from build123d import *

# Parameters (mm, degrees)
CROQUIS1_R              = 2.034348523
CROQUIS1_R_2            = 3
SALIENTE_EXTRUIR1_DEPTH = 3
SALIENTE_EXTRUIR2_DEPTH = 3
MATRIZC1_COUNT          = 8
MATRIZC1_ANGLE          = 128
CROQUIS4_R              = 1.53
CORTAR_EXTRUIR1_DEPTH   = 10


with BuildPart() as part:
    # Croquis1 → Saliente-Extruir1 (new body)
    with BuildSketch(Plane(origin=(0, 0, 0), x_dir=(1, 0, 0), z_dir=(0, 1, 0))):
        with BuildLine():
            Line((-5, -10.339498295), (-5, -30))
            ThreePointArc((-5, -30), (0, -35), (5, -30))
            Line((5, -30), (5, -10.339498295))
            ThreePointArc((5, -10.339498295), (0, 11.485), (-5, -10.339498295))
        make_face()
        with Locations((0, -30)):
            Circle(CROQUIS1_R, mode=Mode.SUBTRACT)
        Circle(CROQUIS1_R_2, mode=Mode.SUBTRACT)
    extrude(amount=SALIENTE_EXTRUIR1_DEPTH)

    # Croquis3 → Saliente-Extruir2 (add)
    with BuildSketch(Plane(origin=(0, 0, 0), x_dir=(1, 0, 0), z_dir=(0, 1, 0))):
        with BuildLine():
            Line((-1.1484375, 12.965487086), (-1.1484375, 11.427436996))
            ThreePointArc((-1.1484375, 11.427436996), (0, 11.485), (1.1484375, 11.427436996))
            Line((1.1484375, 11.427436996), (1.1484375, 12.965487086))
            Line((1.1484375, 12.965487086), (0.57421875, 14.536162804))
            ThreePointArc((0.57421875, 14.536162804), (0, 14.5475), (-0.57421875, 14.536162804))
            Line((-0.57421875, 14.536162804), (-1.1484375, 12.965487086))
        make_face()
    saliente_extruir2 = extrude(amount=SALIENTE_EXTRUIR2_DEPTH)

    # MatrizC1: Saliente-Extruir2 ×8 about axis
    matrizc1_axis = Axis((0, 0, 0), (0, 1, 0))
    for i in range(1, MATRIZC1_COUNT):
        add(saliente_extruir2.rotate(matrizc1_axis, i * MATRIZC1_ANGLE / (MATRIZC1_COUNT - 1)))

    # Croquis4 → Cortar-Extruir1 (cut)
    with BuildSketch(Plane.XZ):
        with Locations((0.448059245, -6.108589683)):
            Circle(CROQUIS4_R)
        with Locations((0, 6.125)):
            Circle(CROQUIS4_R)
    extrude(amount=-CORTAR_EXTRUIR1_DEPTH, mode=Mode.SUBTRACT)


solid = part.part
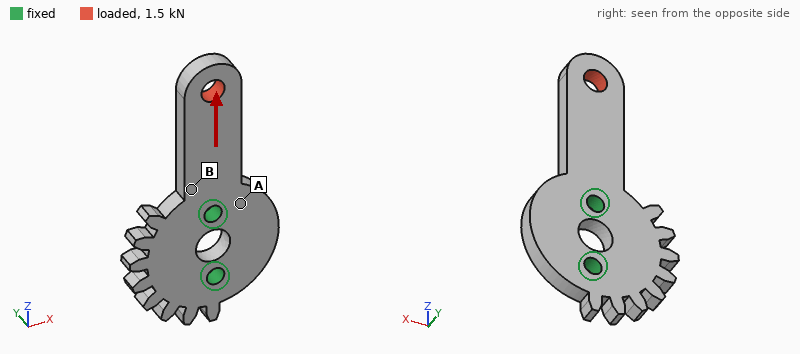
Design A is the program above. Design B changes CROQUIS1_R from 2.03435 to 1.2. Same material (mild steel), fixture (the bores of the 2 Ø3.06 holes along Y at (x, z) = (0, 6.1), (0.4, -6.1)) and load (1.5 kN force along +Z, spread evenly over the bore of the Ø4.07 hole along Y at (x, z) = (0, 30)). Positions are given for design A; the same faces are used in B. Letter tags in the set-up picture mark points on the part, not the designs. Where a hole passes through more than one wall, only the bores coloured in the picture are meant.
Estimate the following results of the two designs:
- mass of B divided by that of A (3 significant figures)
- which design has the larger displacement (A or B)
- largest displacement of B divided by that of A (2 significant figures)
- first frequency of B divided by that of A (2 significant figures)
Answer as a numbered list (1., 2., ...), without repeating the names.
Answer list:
1. 1.01
2. A
3. 0.91
4. 0.96
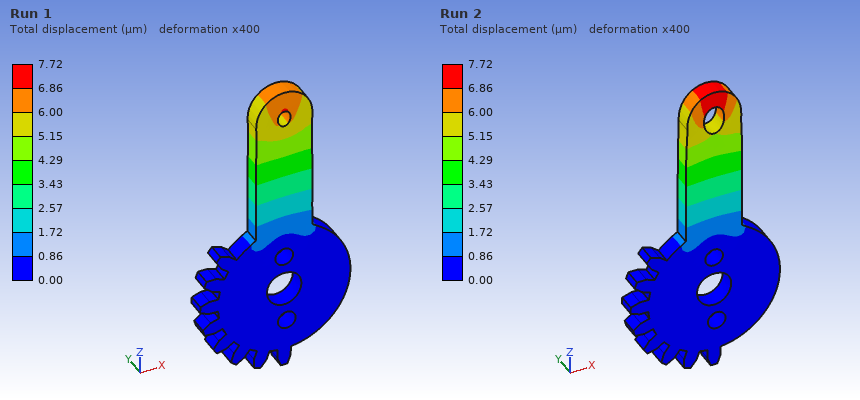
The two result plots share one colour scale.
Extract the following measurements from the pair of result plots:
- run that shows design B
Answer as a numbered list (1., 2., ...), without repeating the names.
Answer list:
1. Run 1
